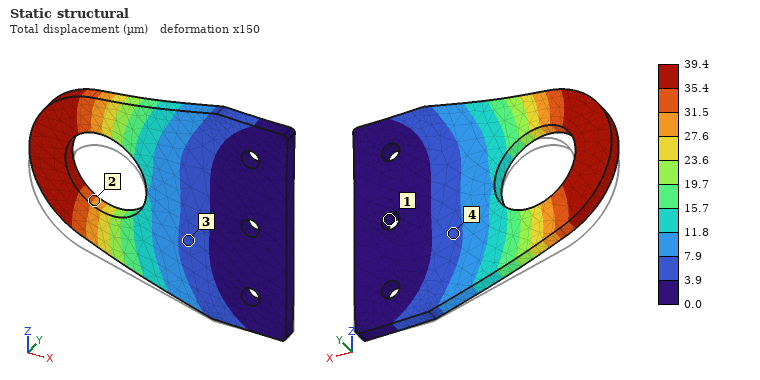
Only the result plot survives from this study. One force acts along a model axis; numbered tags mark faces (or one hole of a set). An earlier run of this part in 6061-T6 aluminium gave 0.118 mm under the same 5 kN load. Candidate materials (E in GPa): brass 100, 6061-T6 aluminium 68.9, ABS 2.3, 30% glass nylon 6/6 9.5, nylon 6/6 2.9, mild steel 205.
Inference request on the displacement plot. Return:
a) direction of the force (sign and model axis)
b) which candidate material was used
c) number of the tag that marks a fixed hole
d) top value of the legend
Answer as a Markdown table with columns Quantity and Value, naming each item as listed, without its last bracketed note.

| Quantity | Value |
|---|---|
| direction of the force | +Z |
| which candidate material was used | mild steel |
| number of the tag that marks a fixed hole | 1 |
| top value of the legend | 39.4 µm |
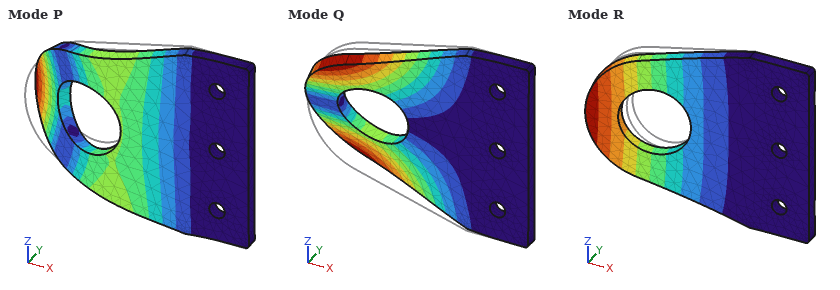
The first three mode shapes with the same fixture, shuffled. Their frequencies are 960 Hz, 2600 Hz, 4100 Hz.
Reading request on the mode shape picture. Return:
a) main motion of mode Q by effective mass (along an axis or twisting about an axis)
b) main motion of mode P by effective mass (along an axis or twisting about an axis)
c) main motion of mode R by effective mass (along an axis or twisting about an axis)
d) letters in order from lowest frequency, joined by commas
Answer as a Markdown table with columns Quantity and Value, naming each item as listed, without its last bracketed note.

| Quantity | Value |
|---|---|
| main motion of mode Q by effective mass | twisting about X |
| main motion of mode P by effective mass | along Y |
| main motion of mode R by effective mass | along Y |
| letters in order from lowest frequency, joined by commas | R, Q, P |
